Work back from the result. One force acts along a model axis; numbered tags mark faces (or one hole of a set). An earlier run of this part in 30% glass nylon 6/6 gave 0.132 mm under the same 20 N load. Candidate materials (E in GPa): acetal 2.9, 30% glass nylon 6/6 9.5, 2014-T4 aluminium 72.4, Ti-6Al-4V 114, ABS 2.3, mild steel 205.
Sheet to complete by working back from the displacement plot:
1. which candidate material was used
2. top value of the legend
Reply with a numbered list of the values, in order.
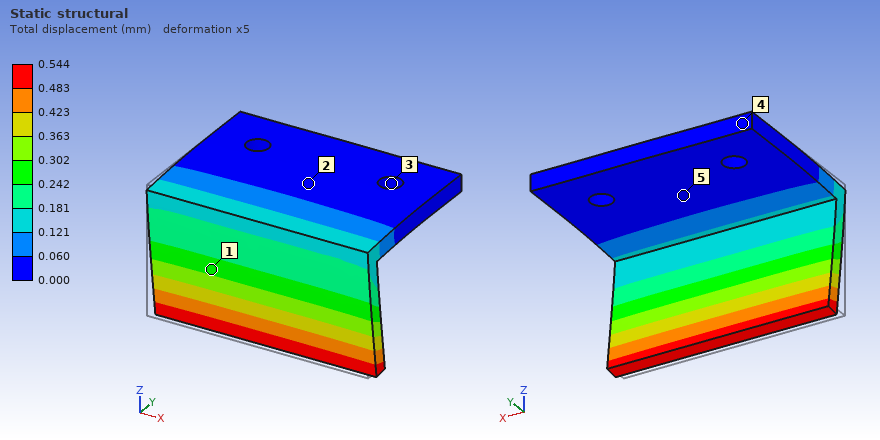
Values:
1. ABS
2. 0.544 mm
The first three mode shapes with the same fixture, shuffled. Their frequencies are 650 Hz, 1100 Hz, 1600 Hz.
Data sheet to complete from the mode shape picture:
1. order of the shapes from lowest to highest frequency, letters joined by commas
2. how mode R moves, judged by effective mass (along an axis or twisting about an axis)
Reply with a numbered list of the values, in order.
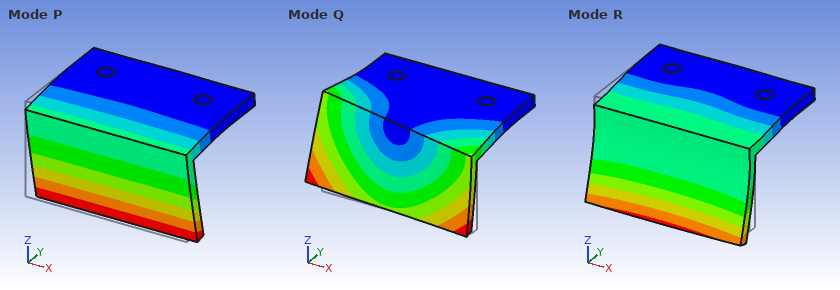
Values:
1. P, Q, R
2. along Z
